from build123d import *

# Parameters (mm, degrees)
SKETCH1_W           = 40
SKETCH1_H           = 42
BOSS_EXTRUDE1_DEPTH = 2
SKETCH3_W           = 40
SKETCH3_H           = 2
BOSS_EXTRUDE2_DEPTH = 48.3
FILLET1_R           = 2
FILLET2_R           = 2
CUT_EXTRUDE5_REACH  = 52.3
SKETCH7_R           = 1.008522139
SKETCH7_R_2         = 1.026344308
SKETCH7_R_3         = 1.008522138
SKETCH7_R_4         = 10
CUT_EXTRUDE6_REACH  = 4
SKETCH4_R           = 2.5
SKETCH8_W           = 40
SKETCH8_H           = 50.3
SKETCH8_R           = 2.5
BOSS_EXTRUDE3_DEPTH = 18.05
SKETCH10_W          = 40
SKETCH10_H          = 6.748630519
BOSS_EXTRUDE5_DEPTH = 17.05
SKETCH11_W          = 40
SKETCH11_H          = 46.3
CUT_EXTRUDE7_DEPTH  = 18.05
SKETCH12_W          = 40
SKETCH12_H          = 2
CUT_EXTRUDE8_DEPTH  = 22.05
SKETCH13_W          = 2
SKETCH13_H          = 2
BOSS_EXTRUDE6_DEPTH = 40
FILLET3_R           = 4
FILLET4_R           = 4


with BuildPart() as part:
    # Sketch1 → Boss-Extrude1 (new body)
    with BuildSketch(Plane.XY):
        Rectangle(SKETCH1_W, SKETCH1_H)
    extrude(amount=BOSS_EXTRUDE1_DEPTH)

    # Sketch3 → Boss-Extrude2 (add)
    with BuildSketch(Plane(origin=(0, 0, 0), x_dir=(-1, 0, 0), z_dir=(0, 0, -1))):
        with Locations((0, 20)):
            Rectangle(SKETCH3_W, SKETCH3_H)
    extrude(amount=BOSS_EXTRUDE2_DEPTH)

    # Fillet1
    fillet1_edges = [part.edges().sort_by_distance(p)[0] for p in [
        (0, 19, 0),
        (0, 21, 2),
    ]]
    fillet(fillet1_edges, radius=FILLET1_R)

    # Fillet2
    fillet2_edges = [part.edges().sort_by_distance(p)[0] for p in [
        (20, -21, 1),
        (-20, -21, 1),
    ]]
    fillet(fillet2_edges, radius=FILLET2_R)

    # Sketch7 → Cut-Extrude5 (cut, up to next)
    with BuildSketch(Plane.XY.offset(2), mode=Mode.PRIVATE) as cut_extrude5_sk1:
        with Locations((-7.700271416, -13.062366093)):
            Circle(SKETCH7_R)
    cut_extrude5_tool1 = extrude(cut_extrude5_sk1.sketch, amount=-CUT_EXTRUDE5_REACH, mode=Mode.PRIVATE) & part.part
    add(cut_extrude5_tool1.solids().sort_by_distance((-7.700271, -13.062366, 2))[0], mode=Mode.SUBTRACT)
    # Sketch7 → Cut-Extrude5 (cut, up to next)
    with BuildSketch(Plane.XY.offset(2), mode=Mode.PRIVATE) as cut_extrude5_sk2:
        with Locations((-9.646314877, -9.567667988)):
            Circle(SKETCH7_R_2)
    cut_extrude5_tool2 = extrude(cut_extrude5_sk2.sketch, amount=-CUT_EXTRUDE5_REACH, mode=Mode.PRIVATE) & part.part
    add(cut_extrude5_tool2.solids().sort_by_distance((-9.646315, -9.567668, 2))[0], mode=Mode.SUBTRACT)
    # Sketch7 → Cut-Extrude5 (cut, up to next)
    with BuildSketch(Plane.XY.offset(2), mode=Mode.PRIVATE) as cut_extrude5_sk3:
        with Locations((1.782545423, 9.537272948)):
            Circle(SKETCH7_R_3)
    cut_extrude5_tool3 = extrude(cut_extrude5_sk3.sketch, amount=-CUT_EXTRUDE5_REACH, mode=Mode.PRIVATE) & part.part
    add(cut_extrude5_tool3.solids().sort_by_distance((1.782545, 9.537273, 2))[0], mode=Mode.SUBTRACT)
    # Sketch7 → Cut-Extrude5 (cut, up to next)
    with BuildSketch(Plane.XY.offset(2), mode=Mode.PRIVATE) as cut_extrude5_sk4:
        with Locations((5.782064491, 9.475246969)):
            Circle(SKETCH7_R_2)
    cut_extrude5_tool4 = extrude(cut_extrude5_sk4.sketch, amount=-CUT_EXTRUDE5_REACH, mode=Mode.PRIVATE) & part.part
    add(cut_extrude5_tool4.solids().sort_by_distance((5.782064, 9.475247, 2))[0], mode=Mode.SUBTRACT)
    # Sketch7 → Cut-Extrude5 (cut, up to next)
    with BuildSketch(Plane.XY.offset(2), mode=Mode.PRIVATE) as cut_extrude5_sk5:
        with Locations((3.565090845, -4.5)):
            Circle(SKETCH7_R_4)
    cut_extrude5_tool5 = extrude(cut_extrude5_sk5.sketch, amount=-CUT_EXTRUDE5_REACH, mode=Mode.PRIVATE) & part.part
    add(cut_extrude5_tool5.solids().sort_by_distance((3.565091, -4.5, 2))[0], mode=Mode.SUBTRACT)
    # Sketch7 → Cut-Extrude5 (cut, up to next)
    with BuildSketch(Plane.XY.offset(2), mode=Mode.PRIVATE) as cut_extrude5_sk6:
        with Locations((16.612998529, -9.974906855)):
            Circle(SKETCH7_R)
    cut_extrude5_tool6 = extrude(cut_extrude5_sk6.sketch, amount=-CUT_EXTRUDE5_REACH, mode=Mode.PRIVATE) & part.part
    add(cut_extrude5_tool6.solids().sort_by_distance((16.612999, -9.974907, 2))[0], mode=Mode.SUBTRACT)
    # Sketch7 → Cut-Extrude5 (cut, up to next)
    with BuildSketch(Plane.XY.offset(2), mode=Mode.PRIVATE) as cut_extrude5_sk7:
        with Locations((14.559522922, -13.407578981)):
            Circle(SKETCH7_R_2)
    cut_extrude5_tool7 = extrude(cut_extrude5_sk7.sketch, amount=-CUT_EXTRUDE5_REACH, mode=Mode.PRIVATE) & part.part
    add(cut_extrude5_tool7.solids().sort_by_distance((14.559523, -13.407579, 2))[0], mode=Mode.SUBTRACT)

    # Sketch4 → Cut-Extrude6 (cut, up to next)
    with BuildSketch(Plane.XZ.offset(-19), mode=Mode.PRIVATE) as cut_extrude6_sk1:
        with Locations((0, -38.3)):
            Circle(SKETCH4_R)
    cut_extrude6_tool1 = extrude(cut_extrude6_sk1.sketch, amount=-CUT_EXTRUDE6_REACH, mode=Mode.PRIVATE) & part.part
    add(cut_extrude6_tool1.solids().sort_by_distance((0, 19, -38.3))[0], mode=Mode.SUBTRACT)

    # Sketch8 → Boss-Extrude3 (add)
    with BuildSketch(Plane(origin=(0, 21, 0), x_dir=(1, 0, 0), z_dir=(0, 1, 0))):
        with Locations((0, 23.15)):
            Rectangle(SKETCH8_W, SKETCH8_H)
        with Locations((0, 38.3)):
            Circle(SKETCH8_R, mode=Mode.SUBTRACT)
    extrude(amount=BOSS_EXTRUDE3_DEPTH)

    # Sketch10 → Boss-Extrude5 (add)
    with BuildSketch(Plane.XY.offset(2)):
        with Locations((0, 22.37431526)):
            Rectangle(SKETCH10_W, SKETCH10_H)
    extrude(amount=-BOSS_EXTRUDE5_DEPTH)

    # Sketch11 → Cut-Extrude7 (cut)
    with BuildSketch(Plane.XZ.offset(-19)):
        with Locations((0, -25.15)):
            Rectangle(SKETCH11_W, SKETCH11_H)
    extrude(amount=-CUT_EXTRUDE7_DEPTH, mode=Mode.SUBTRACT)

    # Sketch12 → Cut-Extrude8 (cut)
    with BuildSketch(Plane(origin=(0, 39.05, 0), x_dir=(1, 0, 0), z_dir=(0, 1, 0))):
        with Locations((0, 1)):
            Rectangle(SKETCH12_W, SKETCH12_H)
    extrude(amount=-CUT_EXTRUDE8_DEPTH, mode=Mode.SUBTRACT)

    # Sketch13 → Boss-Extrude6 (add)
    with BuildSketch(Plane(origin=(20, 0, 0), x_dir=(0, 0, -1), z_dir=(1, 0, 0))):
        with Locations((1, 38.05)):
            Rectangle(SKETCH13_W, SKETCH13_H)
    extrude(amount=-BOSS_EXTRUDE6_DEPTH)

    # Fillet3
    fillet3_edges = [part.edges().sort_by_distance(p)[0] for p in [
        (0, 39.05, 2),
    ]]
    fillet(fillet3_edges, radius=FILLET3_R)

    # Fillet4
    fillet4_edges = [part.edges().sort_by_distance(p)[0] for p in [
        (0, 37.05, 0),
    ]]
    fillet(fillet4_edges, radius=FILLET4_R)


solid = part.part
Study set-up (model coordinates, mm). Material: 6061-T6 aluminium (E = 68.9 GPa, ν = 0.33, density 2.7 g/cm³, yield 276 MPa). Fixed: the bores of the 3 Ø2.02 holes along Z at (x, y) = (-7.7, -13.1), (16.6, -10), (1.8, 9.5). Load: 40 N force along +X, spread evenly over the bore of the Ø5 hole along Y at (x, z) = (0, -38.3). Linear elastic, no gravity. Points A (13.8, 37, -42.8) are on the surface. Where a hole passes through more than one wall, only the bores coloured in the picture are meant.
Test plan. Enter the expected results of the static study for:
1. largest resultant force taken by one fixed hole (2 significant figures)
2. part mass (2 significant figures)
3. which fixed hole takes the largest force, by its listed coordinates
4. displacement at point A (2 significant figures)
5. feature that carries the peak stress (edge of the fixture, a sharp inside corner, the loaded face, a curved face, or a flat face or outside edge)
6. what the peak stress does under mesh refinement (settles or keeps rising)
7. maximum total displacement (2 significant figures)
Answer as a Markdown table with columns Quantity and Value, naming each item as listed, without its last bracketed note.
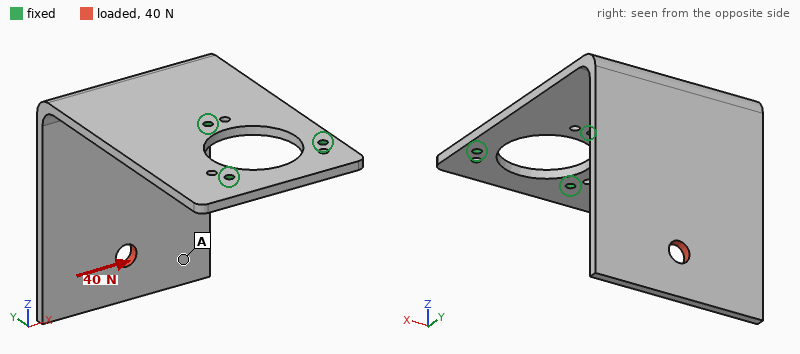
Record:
| Quantity | Value |
|---|---|
| largest resultant force taken by one fixed hole | 54 N |
| part mass | 21 g |
| which fixed hole takes the largest force, by its listed coordinates | (1.8, 9.5) |
| displacement at point A | 0.75 mm |
| feature that carries the peak stress | edge of the fixture |
| what the peak stress does under mesh refinement | keeps rising |
| maximum total displacement | 0.89 mm |
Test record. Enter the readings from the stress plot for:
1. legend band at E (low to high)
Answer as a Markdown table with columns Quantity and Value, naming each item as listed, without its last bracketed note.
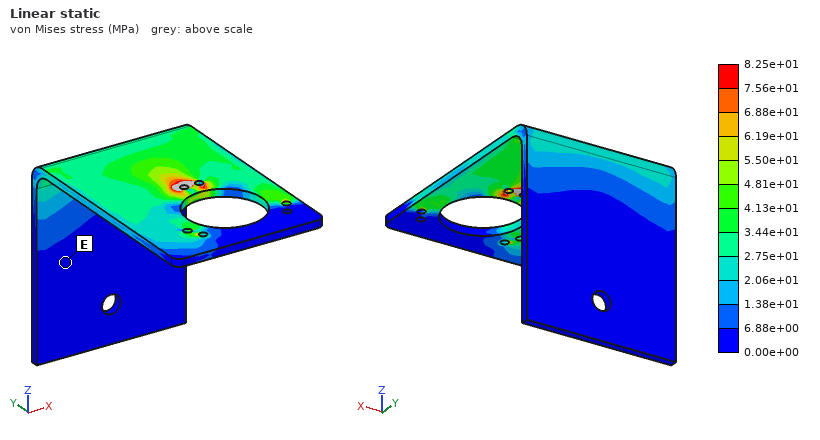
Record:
| Quantity | Value |
|---|---|
| legend band at E | 0.00e+00 to 6.88e+00 MPa |
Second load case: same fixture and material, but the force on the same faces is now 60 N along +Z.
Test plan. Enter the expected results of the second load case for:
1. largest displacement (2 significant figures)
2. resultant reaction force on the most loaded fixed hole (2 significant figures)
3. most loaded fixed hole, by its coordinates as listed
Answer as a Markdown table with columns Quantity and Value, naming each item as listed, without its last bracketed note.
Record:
| Quantity | Value |
|---|---|
| largest displacement | 0.82 mm |
| resultant reaction force on the most loaded fixed hole | 100 N |
| most loaded fixed hole, by its coordinates as listed | (1.8, 9.5) |
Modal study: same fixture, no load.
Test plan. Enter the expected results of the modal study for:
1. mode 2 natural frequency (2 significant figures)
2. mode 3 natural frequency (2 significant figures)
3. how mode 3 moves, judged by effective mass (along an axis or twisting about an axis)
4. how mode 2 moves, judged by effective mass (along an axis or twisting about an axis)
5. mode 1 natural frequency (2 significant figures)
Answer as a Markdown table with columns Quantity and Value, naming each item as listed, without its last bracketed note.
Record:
| Quantity | Value |
|---|---|
| mode 2 natural frequency | 480 Hz |
| mode 3 natural frequency | 1100 Hz |
| how mode 3 moves, judged by effective mass | along Z |
| how mode 2 moves, judged by effective mass | along X |
| mode 1 natural frequency | 350 Hz |
